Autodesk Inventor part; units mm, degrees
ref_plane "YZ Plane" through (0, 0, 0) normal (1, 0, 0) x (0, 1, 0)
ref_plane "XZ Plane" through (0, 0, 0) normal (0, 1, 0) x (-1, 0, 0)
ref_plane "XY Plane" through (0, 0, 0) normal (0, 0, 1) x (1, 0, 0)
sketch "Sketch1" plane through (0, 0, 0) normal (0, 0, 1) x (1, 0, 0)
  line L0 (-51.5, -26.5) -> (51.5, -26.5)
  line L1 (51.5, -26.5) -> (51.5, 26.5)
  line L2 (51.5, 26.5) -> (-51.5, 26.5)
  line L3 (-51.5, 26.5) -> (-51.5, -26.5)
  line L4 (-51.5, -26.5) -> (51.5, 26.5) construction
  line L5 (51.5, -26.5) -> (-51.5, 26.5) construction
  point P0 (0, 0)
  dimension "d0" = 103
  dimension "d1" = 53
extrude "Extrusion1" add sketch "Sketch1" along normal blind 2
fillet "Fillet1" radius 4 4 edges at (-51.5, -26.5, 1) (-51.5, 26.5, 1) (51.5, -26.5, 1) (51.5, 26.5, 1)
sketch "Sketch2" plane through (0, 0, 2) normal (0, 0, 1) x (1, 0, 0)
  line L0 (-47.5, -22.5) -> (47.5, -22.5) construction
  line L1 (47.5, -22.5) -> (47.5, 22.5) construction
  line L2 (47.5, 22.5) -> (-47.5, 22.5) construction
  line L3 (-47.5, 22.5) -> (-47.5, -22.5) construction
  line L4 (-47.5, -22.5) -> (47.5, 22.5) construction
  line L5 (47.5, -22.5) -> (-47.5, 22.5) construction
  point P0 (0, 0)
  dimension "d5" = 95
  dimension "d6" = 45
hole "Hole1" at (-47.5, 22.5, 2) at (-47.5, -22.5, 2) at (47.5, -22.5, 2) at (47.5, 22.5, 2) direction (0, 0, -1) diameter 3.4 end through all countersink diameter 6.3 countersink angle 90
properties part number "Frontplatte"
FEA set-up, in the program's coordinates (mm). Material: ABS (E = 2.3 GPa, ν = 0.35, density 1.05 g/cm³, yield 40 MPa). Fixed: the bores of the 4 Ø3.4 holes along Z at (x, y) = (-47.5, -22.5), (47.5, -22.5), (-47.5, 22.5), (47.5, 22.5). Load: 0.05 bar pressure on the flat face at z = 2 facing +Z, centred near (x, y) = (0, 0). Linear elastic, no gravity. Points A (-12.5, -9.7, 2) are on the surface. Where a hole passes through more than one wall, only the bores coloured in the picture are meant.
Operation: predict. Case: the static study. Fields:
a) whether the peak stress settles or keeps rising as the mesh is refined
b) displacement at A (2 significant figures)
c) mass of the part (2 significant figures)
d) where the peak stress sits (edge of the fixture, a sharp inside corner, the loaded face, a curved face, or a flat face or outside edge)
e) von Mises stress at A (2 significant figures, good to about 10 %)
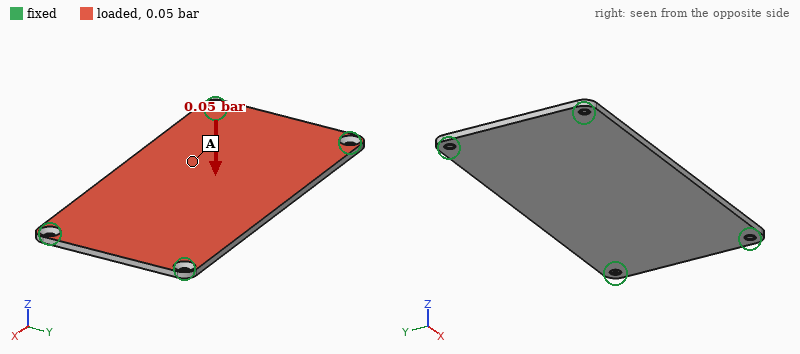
keeps rising
1.0 mm
11 g
edge of the fixture
3.3 MPa
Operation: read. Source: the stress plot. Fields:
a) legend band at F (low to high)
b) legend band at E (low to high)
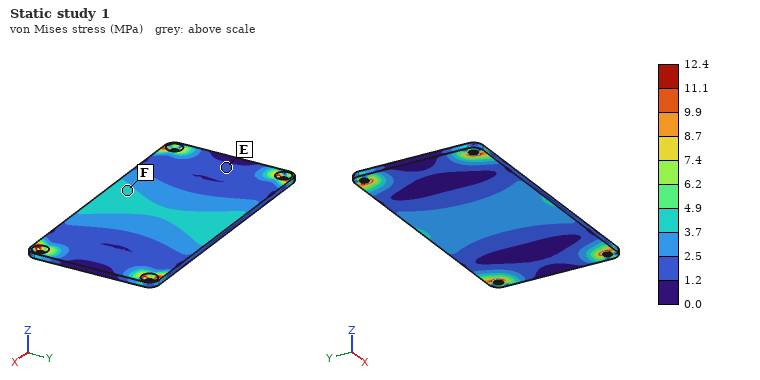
3.7 to 4.9 MPa
1.2 to 2.5 MPa
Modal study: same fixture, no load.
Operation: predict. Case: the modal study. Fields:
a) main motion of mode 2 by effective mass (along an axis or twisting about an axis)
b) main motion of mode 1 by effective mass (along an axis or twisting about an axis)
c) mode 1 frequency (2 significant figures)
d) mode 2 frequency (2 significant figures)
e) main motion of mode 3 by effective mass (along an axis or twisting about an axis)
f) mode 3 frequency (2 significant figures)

twisting about X
along Z
260 Hz
480 Hz
twisting about Y
730 Hz
